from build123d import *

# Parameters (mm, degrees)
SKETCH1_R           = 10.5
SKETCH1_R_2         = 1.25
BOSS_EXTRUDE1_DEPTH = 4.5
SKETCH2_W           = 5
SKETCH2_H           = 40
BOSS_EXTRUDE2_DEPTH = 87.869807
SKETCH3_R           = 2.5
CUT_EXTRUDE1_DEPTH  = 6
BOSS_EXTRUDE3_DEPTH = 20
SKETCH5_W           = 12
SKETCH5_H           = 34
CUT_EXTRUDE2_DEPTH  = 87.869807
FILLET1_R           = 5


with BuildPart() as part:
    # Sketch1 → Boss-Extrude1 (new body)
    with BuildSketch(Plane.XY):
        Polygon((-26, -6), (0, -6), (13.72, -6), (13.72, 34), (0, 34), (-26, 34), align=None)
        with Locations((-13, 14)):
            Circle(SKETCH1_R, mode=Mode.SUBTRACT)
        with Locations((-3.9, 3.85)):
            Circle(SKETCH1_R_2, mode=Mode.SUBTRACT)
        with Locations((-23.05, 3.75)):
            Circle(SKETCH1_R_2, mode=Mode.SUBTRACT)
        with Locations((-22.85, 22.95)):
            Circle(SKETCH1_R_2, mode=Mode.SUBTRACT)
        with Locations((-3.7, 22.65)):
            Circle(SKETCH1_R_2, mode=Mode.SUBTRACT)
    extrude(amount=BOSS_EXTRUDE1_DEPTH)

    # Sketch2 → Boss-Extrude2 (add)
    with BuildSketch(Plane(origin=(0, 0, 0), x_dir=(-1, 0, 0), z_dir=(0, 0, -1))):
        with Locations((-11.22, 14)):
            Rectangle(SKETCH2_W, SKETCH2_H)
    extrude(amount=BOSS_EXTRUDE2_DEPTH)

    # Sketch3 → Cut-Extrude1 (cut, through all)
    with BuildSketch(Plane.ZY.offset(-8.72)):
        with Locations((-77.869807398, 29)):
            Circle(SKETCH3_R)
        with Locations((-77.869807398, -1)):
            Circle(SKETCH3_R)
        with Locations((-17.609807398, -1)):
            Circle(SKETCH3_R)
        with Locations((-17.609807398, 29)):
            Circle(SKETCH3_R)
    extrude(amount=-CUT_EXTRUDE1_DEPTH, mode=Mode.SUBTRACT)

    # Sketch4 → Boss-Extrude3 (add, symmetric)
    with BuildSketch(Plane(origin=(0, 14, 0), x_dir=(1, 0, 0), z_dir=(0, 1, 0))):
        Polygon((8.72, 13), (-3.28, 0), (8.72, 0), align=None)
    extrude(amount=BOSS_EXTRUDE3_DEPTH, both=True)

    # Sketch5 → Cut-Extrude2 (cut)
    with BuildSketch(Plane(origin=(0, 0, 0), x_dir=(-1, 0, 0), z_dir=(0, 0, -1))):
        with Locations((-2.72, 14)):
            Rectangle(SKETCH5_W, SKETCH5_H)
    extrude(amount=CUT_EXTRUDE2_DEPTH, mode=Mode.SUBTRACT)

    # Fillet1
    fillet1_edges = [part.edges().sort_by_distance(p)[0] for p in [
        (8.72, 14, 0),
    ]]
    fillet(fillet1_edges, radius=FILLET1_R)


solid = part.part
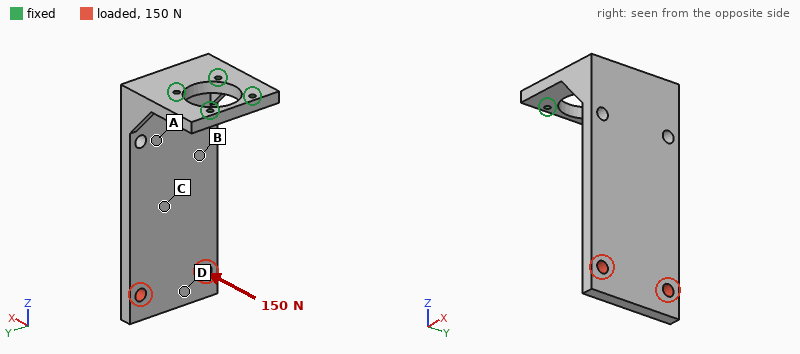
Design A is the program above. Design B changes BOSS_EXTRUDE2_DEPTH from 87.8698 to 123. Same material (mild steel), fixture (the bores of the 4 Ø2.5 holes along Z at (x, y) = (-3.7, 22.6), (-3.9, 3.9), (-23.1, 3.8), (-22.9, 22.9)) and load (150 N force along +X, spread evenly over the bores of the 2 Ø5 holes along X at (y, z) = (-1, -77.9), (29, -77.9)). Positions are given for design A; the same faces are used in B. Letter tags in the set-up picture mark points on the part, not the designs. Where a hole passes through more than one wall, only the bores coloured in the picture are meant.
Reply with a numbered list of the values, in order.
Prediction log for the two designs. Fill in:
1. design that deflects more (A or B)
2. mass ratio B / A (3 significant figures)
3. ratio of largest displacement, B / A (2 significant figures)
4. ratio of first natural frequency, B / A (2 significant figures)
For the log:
1. A
2. 1.30
3. 0.86
4. 0.54
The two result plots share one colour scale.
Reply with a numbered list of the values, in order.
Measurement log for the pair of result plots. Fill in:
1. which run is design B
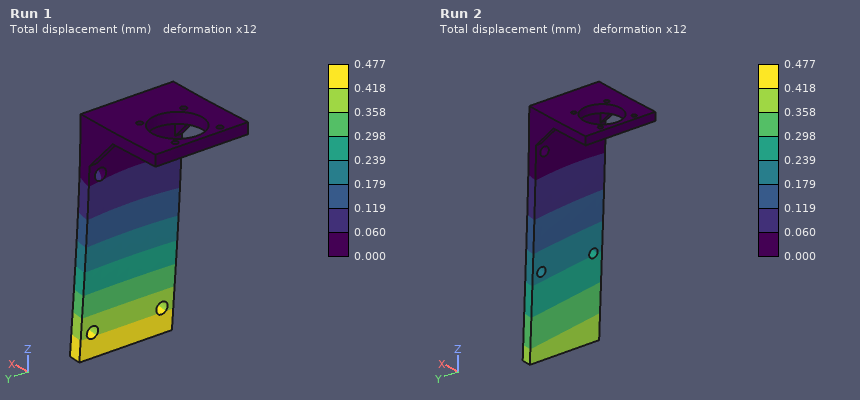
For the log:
1. Run 2
